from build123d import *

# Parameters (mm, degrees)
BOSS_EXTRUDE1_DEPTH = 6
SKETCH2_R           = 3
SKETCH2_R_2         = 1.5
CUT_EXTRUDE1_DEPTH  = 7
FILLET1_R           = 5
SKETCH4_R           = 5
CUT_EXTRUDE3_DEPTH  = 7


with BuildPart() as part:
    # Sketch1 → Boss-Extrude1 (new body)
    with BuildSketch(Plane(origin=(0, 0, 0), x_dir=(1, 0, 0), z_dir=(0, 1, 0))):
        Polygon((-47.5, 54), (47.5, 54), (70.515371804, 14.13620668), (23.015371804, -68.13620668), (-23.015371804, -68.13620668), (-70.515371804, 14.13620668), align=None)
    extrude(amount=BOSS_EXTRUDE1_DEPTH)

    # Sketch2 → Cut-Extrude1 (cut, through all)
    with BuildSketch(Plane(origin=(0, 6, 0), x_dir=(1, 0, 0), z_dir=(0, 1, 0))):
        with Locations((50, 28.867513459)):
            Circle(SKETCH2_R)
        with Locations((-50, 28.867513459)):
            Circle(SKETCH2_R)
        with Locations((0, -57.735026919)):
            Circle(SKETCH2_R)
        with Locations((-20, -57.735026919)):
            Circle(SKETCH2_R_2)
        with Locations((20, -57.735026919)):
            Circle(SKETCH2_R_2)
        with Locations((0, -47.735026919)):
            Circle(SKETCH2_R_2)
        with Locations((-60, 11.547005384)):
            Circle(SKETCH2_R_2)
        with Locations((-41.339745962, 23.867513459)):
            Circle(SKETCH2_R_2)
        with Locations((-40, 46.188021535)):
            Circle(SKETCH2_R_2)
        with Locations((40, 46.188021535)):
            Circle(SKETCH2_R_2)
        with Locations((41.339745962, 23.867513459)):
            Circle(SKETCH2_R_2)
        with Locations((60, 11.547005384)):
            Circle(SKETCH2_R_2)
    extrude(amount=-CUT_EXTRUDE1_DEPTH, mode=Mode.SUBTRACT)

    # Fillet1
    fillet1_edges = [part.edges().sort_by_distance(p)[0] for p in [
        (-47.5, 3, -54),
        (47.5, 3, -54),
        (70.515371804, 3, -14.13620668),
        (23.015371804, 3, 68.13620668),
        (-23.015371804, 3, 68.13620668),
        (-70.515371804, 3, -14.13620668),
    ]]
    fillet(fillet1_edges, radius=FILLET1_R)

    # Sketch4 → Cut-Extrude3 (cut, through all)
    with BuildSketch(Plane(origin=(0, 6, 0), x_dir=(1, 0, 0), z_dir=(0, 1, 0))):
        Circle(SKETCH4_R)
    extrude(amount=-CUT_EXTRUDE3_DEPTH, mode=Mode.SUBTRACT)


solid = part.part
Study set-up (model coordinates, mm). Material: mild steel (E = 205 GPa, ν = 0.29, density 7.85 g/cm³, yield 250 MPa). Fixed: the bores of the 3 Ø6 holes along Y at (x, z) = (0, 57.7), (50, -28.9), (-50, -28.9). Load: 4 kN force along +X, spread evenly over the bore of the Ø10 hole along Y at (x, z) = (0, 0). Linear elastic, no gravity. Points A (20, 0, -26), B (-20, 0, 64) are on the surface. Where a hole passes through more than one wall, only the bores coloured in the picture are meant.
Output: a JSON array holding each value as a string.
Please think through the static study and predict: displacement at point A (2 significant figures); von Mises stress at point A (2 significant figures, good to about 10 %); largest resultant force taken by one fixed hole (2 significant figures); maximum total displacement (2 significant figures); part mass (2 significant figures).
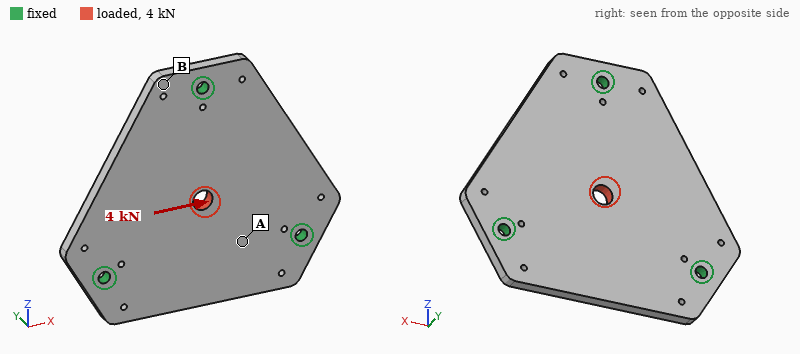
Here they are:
["1.3 µm", "6.9 MPa", "1.5 kN", "3.7 µm", "570 g"]
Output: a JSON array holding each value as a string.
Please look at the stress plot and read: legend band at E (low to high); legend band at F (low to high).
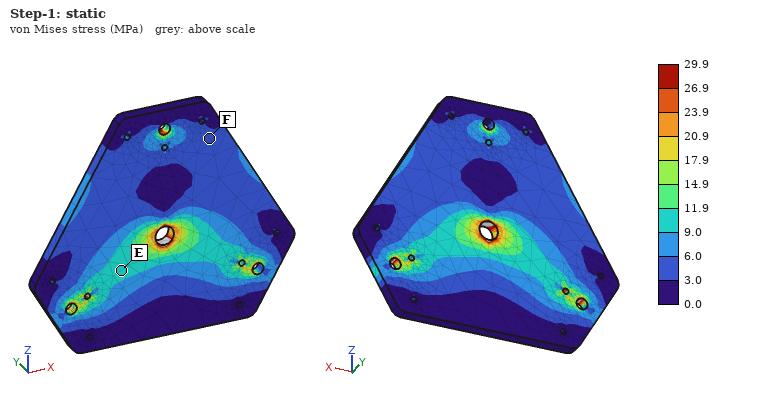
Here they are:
["9.0 to 11.9 MPa", "3.0 to 6.0 MPa"]
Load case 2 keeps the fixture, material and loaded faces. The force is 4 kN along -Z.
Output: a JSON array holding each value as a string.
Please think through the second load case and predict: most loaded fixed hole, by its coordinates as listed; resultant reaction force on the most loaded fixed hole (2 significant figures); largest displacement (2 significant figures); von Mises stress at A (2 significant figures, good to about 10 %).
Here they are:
["(0, 57.7)", "1.6 kN", "3.7 µm", "5.6 MPa"]
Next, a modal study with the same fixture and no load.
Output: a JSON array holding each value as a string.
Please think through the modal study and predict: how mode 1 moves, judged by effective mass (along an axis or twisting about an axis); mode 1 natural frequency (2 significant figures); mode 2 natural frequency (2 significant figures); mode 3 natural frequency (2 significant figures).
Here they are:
["along Y", "2600 Hz", "2900 Hz", "2900 Hz"]
